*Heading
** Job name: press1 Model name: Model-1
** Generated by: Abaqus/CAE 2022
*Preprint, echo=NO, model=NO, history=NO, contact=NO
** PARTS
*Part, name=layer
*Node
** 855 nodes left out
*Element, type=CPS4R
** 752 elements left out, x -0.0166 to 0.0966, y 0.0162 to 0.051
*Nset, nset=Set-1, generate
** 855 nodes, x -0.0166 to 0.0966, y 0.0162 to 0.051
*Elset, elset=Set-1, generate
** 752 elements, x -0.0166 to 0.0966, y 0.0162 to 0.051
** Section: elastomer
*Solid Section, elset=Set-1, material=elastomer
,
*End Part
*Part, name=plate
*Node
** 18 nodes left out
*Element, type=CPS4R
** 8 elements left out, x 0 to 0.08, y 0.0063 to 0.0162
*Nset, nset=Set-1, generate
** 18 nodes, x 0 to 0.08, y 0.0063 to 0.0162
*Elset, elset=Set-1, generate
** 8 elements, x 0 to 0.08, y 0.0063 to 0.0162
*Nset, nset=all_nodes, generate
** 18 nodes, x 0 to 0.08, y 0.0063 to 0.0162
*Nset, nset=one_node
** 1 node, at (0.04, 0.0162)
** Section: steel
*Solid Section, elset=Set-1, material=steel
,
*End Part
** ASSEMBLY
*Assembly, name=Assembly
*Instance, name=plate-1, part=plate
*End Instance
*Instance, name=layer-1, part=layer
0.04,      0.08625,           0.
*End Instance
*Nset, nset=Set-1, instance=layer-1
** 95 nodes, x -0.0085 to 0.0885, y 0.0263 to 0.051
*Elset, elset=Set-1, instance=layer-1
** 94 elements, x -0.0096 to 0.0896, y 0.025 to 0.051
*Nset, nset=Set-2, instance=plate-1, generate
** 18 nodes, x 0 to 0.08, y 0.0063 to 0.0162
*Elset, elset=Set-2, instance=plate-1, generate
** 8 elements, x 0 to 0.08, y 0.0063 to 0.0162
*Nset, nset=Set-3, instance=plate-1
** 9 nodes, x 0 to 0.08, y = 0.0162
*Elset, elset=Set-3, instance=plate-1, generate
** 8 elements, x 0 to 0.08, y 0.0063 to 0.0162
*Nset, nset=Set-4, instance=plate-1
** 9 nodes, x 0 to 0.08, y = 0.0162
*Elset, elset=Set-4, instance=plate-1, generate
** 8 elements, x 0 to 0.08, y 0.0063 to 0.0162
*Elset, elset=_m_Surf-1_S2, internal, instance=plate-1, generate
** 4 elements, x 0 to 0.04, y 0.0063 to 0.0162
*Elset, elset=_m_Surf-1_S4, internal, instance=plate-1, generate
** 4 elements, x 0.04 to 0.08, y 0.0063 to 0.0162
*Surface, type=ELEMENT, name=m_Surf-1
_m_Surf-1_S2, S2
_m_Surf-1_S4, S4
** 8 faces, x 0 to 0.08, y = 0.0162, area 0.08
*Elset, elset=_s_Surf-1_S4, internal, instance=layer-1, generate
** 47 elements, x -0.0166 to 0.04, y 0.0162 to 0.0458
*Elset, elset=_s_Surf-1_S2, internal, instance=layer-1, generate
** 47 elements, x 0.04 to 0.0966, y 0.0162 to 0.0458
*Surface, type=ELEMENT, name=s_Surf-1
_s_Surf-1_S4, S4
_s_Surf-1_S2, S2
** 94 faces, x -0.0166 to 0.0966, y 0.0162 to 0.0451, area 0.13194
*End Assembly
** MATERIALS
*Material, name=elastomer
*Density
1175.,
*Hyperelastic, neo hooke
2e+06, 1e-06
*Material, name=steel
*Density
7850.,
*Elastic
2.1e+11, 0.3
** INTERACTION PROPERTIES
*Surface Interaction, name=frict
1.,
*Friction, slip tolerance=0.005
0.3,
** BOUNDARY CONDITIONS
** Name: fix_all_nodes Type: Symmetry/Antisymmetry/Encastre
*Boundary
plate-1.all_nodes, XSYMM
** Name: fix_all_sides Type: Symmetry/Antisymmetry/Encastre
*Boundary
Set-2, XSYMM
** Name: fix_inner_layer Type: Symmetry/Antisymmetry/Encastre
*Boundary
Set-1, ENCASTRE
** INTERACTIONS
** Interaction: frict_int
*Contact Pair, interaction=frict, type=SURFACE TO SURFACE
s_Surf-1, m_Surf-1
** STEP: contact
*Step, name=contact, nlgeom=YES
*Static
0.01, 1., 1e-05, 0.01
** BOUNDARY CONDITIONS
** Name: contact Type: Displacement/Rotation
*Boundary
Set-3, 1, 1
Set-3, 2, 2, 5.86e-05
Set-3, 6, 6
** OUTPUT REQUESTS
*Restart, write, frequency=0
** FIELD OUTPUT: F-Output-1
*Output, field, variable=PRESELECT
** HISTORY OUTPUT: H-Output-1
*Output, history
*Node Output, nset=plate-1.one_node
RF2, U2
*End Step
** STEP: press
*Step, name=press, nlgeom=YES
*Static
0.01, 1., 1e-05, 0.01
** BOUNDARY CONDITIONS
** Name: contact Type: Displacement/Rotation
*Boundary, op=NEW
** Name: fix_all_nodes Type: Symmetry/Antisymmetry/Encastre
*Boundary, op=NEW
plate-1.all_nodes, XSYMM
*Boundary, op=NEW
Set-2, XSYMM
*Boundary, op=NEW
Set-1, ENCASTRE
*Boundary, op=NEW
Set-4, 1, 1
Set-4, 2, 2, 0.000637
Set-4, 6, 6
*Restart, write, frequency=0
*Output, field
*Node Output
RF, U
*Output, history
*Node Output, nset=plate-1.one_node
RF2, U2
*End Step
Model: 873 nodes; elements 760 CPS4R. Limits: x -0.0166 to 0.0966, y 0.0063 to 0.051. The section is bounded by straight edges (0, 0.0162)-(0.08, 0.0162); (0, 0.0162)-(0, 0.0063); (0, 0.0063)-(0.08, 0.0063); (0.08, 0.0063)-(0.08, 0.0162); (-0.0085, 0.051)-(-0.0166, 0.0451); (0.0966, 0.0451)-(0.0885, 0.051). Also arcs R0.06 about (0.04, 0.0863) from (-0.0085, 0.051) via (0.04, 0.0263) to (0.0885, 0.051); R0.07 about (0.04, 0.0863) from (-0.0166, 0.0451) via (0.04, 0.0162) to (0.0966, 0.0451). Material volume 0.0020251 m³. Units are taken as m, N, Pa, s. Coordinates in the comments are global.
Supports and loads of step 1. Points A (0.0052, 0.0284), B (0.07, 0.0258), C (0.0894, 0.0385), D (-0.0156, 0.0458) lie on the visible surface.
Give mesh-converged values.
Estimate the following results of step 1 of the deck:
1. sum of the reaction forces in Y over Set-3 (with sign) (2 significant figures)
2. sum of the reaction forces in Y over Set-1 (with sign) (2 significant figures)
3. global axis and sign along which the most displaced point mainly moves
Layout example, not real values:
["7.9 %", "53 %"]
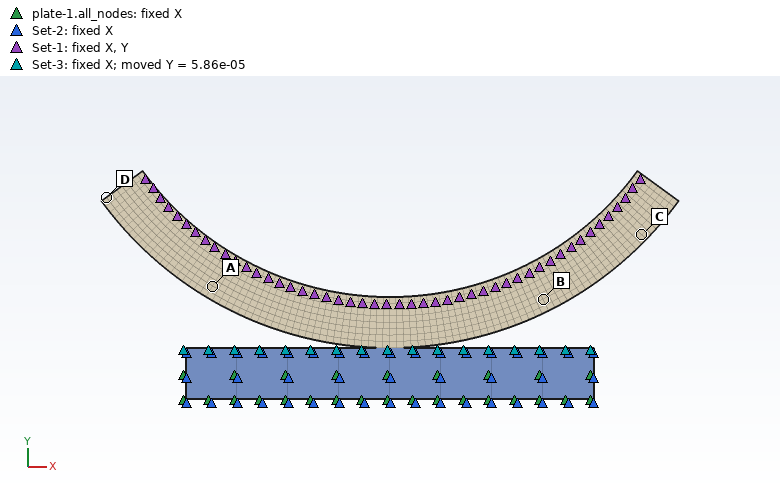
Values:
["260 N", "-260 N", "+Y"]
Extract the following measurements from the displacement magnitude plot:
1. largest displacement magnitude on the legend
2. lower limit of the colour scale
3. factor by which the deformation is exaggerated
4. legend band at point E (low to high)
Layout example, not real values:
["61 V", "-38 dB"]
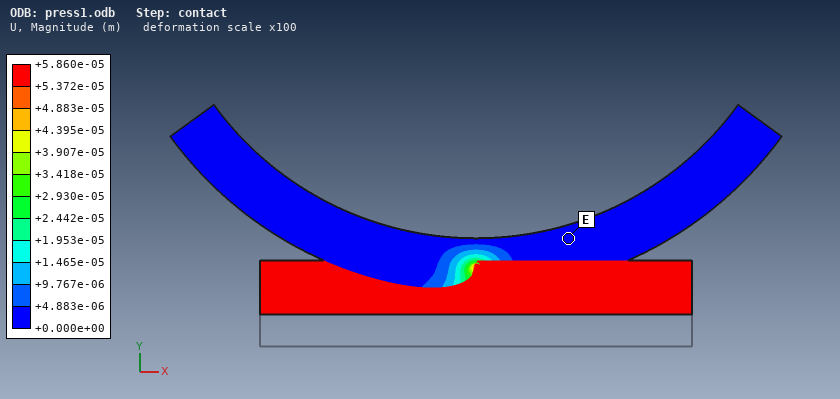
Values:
["+5.860e-05 m", "+0.000e+00 m", "100", "+0.000e+00 to +4.883e-06 m"]
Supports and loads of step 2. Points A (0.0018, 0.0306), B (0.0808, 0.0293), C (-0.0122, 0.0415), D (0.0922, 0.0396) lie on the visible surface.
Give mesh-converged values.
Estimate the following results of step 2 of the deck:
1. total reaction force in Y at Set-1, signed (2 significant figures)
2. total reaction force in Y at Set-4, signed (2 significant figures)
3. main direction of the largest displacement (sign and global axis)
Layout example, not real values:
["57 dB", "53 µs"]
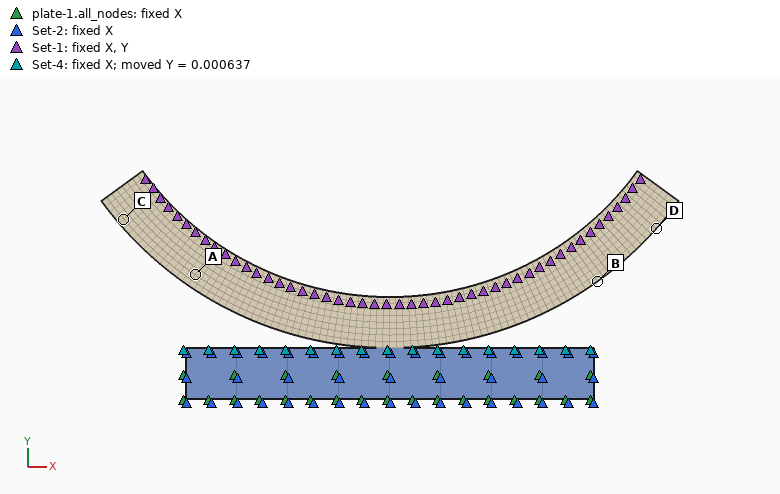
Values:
["-6400 N", "6400 N", "+Y"]
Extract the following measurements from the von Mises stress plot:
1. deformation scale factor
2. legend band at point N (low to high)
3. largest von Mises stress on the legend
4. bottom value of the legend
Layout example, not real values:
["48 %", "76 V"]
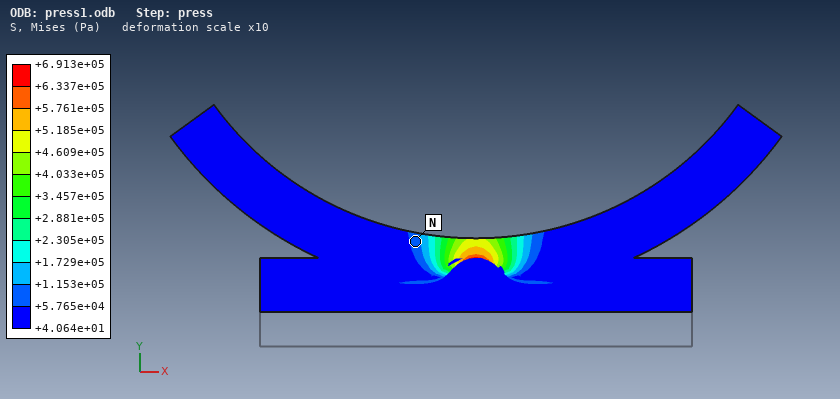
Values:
["10", "+5.765e+04 to +1.153e+05 Pa", "+6.913e+05 Pa", "+4.064e+01 Pa"]
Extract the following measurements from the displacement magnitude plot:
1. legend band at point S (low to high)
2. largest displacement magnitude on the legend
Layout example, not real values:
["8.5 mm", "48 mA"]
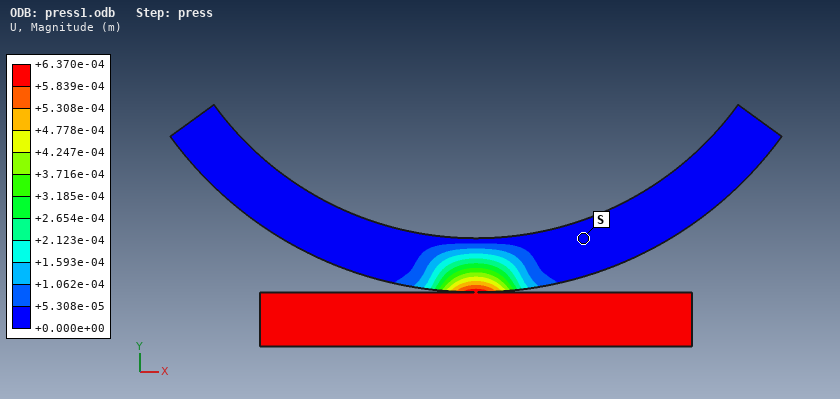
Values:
["+0.000e+00 to +5.308e-05 m", "+6.370e-04 m"]
